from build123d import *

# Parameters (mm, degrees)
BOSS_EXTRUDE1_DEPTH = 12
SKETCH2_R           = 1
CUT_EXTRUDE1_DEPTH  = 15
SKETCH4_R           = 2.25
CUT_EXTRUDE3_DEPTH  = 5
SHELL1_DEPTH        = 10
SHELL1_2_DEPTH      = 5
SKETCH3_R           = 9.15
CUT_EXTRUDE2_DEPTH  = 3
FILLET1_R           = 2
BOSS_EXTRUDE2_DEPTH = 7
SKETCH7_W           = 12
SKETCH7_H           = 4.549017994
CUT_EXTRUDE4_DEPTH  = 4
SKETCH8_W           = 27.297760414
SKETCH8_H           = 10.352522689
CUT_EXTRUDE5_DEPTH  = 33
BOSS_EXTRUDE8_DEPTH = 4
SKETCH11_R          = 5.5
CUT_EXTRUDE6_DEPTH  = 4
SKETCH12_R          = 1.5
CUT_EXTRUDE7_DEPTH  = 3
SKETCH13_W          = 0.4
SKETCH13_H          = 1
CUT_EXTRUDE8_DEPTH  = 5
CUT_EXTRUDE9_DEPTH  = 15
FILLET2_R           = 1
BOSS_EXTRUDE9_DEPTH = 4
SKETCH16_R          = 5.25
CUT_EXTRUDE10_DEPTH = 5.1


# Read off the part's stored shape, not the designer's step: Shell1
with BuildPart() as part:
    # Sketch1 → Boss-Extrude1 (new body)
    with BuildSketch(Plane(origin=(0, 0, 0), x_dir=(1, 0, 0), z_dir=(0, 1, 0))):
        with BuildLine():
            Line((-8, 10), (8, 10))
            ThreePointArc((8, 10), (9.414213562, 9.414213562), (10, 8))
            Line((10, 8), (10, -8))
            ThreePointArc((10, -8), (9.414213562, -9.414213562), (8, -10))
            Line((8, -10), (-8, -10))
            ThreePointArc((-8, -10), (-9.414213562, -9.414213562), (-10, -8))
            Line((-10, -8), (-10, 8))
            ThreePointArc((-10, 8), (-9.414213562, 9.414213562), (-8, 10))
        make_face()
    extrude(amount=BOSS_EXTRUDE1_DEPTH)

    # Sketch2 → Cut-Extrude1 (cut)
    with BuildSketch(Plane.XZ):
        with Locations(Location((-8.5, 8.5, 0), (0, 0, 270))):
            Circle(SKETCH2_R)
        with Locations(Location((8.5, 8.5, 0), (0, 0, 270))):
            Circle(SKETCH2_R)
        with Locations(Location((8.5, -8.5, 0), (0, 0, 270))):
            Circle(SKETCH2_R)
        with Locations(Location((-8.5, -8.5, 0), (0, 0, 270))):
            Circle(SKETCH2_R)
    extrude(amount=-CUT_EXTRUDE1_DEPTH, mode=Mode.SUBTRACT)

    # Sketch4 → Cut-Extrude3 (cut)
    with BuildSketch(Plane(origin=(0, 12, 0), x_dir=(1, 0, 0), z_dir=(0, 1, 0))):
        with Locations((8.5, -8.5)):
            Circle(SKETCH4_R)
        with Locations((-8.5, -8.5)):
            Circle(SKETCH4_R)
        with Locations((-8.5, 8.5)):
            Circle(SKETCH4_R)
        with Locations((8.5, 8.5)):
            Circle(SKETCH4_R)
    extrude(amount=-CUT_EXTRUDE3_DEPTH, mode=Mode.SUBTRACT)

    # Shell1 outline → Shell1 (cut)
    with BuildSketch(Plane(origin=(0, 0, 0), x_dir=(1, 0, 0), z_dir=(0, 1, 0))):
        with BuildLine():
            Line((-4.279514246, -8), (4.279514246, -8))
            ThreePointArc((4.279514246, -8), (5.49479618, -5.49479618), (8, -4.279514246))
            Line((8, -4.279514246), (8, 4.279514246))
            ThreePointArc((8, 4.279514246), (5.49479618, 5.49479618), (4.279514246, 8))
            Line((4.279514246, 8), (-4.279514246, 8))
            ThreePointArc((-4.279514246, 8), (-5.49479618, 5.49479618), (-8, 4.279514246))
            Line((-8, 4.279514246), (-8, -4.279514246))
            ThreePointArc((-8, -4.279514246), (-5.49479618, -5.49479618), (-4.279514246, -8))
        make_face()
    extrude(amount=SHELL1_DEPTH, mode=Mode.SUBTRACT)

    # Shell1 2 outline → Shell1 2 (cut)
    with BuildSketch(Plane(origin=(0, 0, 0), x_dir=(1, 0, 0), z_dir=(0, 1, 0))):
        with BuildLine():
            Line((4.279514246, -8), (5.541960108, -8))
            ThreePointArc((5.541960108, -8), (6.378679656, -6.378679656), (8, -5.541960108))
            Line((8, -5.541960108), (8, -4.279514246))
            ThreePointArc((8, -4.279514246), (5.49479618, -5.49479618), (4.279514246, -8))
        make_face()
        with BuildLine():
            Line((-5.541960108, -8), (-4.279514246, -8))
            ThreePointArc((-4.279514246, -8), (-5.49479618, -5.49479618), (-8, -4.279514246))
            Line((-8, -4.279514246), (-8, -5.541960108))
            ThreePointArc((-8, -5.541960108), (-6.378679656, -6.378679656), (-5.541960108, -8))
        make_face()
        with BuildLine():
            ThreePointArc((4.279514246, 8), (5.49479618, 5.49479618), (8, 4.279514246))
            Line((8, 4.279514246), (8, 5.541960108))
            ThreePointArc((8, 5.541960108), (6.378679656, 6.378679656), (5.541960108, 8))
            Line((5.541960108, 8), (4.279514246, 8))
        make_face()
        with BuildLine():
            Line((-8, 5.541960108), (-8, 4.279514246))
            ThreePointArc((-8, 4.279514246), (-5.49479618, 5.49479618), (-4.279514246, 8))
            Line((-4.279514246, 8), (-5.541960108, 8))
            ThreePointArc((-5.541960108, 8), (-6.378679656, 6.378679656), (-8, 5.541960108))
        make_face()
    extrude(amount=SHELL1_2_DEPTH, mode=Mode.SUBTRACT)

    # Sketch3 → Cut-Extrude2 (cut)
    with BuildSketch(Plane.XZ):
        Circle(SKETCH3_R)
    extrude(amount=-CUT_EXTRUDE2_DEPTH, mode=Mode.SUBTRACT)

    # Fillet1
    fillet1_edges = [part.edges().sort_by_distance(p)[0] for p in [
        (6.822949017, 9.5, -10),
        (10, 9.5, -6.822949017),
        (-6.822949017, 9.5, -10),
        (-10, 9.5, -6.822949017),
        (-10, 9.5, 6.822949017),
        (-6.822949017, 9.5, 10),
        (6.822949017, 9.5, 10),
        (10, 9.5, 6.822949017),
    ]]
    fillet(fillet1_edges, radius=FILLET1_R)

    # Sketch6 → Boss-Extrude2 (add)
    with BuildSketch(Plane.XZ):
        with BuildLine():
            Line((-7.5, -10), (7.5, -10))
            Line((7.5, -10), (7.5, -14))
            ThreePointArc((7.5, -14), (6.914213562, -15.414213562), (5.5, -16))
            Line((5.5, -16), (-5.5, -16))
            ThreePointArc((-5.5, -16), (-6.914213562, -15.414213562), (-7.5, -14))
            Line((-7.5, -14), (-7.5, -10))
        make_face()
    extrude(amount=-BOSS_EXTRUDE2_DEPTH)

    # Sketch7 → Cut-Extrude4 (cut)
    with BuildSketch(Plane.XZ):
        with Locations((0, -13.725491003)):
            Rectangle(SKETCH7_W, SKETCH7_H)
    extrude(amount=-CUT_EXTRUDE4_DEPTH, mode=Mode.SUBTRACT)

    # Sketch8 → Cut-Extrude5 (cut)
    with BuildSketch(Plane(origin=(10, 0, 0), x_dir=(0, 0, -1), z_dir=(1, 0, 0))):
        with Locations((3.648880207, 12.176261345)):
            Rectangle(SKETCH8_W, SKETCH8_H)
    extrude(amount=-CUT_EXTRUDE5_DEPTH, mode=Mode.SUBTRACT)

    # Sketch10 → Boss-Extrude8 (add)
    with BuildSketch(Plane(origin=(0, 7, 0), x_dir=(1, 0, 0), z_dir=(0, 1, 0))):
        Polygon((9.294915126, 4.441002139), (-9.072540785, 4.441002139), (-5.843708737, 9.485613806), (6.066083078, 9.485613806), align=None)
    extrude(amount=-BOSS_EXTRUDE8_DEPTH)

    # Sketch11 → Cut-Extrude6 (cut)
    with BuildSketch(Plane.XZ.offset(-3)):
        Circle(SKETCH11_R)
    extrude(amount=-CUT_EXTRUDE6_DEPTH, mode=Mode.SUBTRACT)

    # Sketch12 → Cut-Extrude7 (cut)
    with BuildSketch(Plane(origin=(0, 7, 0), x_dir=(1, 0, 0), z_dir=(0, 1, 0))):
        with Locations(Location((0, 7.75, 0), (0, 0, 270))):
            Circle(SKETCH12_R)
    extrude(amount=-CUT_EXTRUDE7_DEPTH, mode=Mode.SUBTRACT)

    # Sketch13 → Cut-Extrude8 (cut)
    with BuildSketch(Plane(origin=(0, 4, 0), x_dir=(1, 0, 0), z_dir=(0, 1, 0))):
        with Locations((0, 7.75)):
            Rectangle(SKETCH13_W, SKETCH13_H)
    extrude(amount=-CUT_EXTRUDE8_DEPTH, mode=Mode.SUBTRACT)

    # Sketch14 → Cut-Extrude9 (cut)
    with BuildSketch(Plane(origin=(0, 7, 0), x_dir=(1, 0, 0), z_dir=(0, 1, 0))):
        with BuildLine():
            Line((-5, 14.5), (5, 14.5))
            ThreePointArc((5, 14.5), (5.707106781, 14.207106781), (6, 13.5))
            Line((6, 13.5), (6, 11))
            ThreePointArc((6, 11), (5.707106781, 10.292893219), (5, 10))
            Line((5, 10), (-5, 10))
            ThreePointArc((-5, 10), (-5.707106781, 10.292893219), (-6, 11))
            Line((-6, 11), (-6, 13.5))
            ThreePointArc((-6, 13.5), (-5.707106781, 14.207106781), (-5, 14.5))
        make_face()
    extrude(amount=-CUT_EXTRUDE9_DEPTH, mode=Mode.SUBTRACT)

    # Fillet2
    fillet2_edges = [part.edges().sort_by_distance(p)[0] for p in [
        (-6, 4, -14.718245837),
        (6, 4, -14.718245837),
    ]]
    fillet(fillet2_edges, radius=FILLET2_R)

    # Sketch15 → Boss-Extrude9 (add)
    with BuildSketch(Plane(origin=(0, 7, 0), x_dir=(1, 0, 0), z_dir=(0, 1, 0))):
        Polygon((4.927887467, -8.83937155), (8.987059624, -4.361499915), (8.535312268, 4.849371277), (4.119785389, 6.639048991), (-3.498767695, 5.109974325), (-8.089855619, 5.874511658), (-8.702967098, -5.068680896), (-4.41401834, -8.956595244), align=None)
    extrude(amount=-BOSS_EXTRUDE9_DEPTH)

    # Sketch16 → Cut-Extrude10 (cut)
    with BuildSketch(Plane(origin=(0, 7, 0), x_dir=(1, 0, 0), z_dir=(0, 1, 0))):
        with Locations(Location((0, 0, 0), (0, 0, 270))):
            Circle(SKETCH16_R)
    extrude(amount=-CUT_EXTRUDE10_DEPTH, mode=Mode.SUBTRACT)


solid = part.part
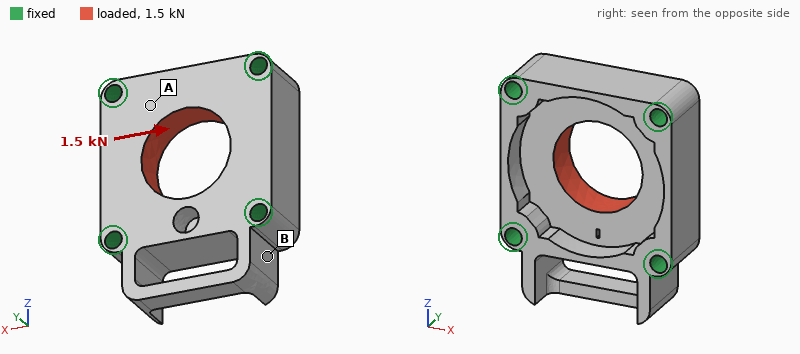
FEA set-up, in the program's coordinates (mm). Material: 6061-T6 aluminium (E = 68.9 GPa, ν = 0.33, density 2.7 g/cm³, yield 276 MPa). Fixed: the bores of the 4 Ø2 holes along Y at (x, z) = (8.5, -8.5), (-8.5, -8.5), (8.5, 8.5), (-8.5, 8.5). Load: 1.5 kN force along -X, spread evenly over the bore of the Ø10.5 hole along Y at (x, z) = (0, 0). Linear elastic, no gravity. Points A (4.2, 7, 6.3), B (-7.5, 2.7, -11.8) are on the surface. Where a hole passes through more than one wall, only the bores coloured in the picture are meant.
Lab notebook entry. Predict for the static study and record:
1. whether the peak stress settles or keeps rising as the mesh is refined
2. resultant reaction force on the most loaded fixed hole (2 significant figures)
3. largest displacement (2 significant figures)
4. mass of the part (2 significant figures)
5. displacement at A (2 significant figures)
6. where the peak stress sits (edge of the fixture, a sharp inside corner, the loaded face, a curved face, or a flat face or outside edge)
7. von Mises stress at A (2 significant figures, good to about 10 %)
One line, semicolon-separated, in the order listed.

keeps rising; 420 N; 4.1 µm; 4.6 g; 1.3 µm; edge of the fixture; 14 MPa
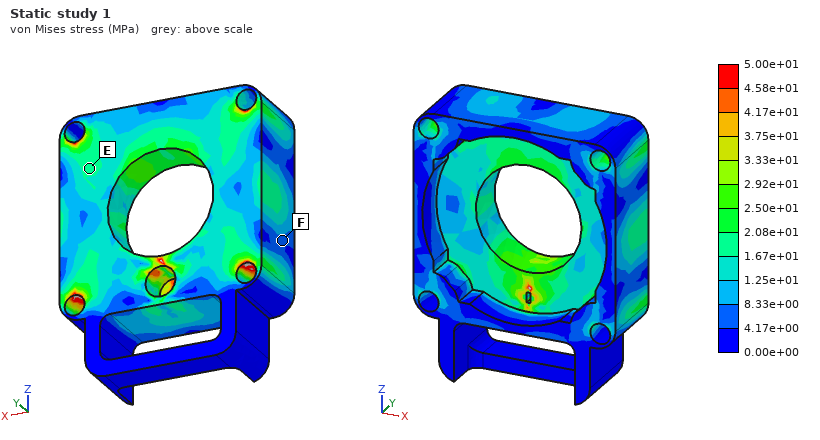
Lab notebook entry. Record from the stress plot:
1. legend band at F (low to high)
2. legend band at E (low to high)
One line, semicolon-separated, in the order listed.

4.17e+00 to 8.33e+00 MPa; 1.67e+01 to 2.08e+01 MPa
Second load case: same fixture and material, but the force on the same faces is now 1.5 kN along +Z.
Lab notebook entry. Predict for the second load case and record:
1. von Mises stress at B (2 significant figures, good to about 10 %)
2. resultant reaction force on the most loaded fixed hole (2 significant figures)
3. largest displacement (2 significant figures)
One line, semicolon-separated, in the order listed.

6.6 MPa; 410 N; 4.4 µm
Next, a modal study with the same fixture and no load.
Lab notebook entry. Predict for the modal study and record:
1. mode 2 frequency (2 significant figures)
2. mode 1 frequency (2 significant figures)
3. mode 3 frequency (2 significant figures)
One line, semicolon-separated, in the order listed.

36 kHz; 29 kHz; 41 kHz
